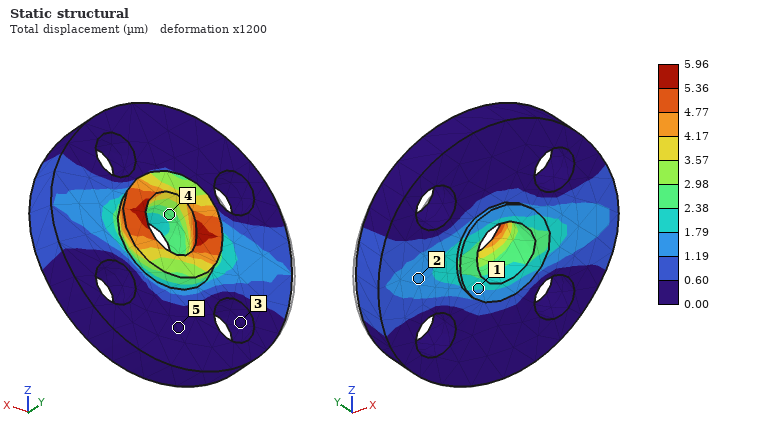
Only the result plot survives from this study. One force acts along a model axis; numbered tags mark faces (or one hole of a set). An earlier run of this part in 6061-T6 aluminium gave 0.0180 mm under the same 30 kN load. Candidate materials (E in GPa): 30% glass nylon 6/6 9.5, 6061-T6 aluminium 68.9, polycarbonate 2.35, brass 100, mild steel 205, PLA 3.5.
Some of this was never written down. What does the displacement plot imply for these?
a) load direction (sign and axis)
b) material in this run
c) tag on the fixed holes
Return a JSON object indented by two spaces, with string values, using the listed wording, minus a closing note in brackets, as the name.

{
  "load direction": "+X",
  "material in this run": "mild steel",
  "tag on the fixed holes": "3"
}
